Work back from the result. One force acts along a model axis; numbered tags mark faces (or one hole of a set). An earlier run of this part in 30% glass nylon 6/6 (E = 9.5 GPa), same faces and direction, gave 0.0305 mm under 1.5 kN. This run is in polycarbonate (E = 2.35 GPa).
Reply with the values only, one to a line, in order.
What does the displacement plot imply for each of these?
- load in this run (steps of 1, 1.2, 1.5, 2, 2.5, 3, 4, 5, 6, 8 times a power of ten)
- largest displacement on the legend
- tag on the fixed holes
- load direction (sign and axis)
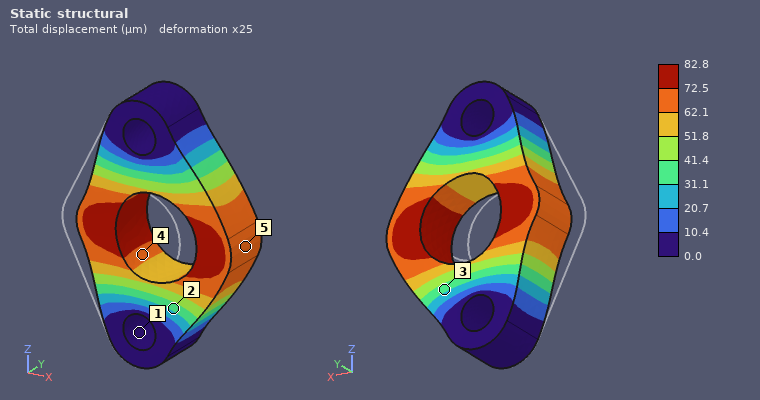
1 kN
82.8 µm
1
+X
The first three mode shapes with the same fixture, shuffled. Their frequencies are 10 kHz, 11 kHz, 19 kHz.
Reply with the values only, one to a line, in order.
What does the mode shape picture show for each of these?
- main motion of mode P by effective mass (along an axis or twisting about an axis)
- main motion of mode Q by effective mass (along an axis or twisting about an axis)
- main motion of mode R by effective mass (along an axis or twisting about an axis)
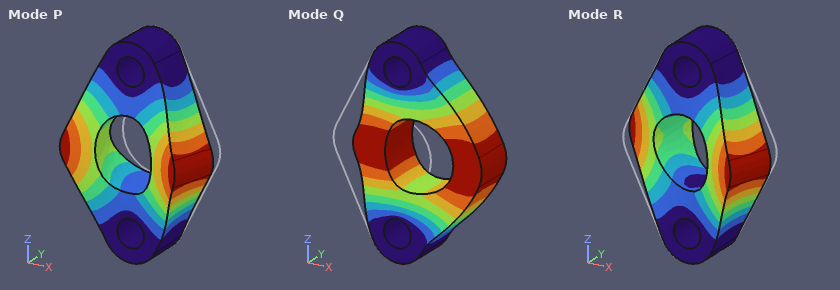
along Y
along X
twisting about Z
